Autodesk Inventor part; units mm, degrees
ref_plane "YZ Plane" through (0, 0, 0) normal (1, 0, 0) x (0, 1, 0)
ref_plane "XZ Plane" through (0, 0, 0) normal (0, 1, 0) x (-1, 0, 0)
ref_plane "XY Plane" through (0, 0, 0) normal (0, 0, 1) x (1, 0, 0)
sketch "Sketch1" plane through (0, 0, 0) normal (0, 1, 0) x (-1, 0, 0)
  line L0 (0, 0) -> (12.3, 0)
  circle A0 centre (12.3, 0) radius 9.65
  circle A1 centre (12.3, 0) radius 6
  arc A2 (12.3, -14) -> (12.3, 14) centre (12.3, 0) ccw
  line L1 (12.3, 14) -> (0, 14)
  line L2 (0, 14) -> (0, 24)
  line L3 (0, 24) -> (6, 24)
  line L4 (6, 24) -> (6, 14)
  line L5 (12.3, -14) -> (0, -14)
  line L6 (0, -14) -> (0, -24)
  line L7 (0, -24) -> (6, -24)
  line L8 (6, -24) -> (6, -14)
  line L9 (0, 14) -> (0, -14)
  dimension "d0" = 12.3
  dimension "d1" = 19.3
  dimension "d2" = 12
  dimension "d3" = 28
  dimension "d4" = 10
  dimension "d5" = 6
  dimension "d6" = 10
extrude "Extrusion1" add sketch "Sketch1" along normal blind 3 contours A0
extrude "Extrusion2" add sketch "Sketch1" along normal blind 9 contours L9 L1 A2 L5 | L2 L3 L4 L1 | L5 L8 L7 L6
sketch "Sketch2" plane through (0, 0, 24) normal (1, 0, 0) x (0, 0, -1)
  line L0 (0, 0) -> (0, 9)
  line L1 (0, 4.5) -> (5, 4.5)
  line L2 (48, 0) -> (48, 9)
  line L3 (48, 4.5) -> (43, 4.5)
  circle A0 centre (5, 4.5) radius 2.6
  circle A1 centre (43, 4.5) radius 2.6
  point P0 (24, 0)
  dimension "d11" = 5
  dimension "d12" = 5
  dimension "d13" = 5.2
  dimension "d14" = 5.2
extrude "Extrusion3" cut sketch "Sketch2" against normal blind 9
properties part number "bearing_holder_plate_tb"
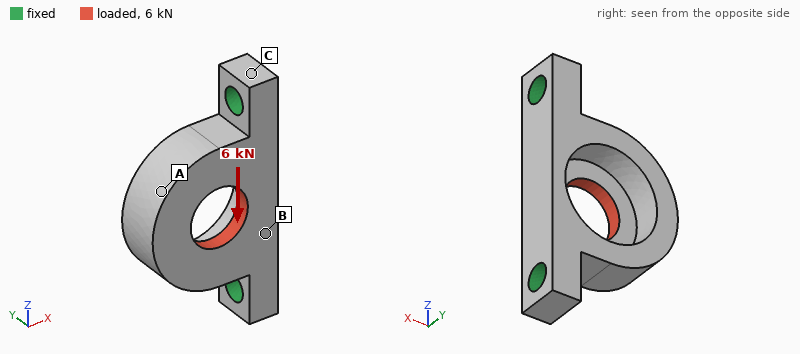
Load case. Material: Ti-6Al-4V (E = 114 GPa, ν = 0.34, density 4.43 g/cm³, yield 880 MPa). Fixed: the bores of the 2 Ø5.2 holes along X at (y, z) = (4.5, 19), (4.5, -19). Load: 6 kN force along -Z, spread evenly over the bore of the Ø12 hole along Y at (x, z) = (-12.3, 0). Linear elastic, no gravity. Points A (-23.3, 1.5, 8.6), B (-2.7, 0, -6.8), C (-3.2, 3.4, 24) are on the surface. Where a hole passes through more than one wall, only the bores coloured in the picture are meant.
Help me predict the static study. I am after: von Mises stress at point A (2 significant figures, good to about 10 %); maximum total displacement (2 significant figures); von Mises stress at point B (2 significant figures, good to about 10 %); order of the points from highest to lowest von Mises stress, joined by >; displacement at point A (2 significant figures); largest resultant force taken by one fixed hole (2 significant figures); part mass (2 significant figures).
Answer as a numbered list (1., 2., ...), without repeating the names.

1. 69 MPa
2. 42 µm
3. 45 MPa
4. A > B > C
5. 38 µm
6. 3.5 kN
7. 20 g
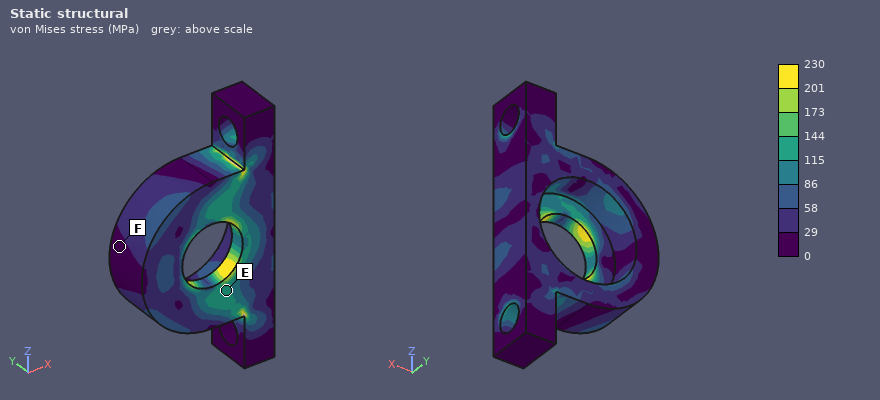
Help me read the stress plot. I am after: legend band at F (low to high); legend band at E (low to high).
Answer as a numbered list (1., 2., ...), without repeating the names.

1. 0 to 29 MPa
2. 115 to 144 MPa
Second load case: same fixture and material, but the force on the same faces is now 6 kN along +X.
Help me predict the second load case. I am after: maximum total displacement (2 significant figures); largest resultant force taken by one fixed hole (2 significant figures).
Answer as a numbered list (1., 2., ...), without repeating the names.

1. 97 µm
2. 3.1 kN
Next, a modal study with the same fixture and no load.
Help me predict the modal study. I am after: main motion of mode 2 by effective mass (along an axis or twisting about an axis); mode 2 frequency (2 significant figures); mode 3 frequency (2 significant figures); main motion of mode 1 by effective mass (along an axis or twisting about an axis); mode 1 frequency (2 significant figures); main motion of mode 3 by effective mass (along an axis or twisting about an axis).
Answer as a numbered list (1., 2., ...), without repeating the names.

1. along Z
2. 15 kHz
3. 21 kHz
4. along Y
5. 7000 Hz
6. along Z
